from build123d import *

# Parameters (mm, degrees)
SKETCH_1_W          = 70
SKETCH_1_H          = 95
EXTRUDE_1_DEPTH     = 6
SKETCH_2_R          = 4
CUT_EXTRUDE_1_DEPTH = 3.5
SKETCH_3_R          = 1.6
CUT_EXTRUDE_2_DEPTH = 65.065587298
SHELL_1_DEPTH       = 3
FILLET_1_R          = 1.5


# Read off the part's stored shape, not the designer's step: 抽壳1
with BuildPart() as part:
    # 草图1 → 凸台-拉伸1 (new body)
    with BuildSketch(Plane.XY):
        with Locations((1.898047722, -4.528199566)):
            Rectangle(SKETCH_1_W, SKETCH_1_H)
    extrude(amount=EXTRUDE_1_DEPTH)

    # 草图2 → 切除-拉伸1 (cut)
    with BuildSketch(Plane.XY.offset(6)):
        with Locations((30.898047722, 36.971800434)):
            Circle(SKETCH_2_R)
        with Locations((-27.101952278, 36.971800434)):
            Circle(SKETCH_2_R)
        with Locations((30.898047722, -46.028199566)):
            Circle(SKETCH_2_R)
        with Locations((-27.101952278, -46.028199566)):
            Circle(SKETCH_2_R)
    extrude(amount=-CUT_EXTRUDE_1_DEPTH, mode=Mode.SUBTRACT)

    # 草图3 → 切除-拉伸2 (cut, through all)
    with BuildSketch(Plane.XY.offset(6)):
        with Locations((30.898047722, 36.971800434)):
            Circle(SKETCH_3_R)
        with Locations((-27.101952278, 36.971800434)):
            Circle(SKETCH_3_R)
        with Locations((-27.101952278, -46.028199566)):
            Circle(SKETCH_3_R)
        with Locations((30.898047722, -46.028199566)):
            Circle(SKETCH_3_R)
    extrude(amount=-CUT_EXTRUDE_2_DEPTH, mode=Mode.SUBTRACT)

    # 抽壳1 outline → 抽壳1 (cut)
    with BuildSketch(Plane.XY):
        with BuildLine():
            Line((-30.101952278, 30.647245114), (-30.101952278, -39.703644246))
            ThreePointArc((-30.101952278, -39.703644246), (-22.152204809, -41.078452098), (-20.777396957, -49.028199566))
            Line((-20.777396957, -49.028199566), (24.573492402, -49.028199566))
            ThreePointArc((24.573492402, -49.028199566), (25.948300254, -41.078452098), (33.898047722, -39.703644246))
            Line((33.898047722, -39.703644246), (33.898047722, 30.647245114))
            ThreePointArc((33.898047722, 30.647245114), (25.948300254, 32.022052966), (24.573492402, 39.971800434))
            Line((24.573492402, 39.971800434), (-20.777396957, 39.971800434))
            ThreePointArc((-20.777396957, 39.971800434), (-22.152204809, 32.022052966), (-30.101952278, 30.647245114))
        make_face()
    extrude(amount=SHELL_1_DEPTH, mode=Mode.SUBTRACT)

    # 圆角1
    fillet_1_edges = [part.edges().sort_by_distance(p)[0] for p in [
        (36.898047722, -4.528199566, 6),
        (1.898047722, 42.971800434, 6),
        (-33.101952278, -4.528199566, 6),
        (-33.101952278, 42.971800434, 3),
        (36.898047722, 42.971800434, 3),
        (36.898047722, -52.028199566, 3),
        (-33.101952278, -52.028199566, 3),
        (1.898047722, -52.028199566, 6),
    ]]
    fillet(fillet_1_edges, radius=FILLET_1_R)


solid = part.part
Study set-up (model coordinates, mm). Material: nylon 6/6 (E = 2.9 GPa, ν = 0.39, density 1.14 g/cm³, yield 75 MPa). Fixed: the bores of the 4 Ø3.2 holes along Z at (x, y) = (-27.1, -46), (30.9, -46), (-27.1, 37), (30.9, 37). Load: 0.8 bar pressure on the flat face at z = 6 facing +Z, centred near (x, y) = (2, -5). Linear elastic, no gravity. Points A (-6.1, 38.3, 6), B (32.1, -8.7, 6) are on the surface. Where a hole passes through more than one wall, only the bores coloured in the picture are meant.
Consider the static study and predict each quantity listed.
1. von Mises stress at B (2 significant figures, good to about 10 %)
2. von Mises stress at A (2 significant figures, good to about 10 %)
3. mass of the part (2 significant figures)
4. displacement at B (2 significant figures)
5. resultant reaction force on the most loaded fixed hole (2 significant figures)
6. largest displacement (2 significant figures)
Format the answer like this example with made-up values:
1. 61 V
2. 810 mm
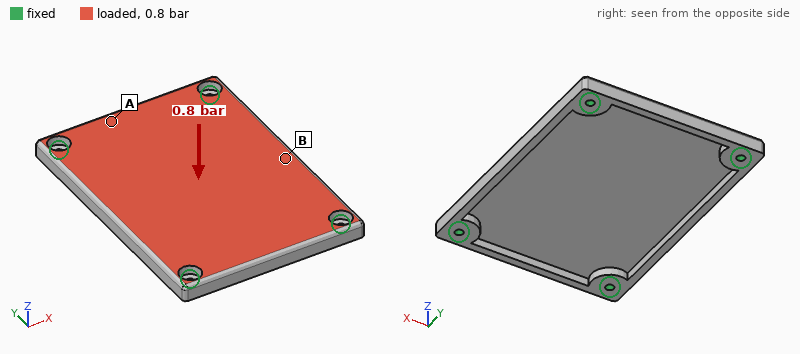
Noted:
1. 12 MPa
2. 5.5 MPa
3. 26 g
4. 0.85 mm
5. 290 N
6. 1.4 mm
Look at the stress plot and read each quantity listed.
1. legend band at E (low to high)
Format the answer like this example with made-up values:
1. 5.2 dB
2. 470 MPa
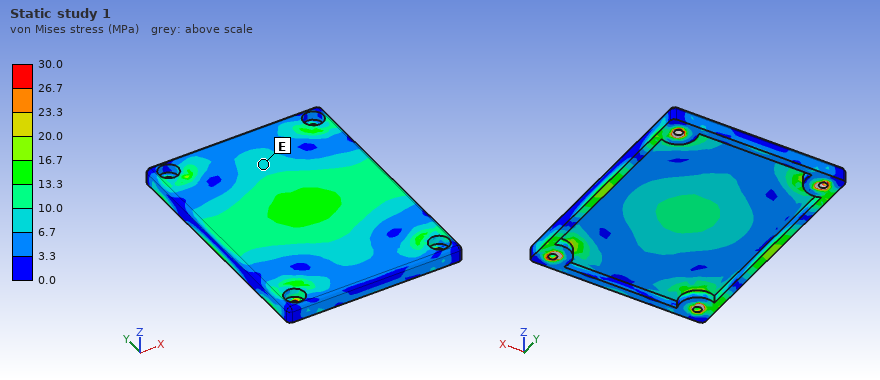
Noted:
1. 6.7 to 10.0 MPa
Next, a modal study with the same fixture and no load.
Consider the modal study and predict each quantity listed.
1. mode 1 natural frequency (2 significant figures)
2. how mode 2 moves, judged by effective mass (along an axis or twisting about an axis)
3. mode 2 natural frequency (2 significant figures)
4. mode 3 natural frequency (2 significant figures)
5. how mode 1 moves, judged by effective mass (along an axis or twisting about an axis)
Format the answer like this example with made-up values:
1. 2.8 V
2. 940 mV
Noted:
1. 770 Hz
2. twisting about Y
3. 1100 Hz
4. 1600 Hz
5. along Z
